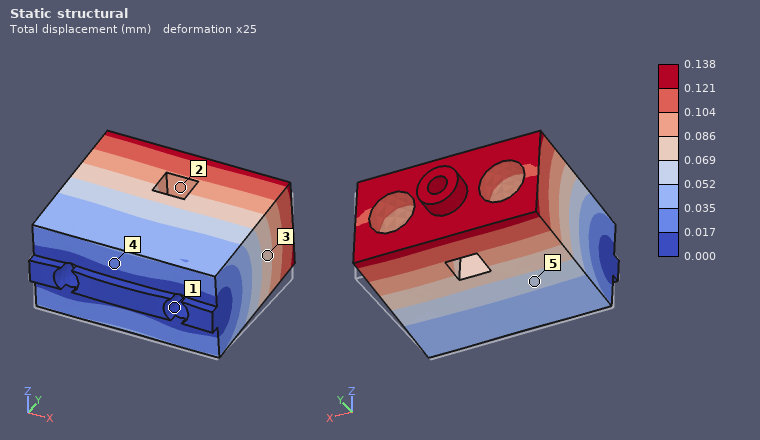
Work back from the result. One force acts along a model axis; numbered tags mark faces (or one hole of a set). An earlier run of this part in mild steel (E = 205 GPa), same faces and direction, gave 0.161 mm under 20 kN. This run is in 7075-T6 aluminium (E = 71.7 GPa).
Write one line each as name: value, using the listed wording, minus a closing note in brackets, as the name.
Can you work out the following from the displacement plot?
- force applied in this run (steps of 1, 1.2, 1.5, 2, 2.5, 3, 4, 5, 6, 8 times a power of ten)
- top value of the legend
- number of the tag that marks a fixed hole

force applied in this run: 6 kN
top value of the legend: 0.138 mm
number of the tag that marks a fixed hole: 1
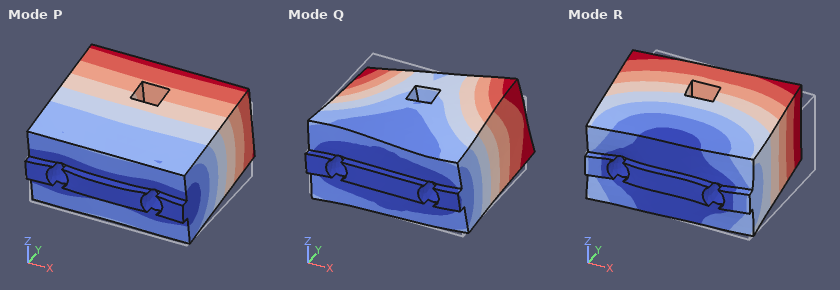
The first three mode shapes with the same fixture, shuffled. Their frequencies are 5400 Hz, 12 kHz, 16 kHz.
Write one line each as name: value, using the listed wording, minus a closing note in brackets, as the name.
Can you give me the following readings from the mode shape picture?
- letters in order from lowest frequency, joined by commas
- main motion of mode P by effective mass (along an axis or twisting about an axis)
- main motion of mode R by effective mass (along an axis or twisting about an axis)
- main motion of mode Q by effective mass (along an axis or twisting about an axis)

letters in order from lowest frequency, joined by commas: P, R, Q
main motion of mode P by effective mass: along Z
main motion of mode R by effective mass: along X
main motion of mode Q by effective mass: twisting about Y
